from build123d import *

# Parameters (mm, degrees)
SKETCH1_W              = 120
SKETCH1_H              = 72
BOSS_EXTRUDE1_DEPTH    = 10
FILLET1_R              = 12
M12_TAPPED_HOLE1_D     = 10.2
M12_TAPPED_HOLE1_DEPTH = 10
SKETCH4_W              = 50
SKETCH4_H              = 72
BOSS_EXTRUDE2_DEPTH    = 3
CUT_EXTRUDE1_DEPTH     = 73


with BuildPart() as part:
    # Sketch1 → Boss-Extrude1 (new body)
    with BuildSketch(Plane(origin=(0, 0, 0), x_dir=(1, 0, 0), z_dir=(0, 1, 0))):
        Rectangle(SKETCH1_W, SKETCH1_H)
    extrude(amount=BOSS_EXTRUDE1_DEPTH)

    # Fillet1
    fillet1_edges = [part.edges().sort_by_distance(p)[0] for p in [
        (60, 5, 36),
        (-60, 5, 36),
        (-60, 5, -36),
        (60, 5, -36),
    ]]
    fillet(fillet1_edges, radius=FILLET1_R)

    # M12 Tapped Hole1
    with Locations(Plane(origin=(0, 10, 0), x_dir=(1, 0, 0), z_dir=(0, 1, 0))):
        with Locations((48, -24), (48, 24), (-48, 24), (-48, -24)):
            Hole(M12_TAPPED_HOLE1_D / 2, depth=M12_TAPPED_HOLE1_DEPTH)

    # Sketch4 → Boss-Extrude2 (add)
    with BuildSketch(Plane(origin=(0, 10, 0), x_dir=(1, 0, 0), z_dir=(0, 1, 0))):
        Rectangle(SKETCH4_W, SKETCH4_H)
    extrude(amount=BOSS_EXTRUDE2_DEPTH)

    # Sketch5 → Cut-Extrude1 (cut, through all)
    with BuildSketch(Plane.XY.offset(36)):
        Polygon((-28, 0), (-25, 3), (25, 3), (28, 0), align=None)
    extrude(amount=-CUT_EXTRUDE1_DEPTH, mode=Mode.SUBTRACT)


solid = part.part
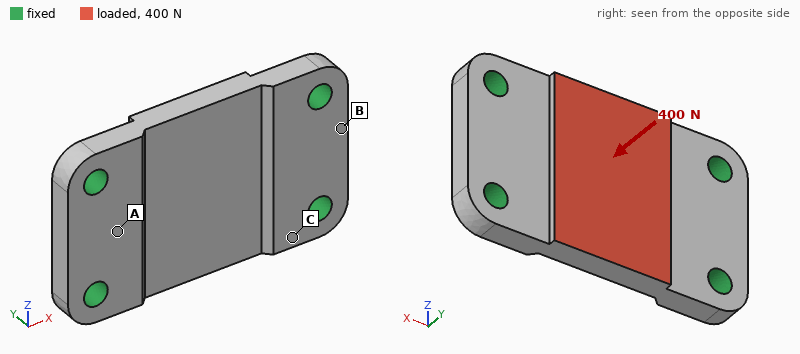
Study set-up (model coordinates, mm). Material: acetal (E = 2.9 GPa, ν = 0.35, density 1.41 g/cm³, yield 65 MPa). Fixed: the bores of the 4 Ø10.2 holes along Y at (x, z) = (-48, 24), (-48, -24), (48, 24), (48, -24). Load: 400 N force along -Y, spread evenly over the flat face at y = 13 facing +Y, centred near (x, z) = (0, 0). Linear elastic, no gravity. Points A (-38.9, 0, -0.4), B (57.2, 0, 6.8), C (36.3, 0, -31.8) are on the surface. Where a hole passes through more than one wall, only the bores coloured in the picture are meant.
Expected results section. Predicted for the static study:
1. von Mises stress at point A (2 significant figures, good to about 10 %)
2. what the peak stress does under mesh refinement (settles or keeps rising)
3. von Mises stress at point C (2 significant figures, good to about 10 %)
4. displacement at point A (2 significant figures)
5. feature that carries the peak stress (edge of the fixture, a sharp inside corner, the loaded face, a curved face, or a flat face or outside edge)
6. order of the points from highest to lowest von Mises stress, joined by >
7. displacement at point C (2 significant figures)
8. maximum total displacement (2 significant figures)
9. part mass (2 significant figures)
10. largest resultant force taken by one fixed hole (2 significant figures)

0.95 MPa
keeps rising
2.0 MPa
18 µm
edge of the fixture
C > A > B
16 µm
79 µm
110 g
160 N
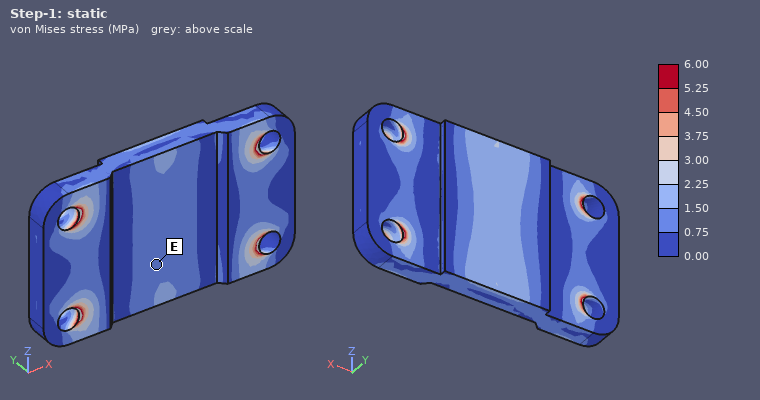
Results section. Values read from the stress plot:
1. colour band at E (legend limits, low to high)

0.75 to 1.50 MPa
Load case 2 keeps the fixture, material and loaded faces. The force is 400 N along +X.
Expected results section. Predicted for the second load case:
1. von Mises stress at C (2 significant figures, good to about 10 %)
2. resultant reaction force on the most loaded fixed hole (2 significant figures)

0.25 MPa
100 N
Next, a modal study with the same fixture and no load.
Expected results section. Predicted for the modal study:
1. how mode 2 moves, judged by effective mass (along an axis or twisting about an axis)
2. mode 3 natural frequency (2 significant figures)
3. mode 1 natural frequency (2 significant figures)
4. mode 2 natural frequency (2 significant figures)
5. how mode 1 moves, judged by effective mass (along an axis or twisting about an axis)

twisting about X
3700 Hz
1700 Hz
2100 Hz
along Y
